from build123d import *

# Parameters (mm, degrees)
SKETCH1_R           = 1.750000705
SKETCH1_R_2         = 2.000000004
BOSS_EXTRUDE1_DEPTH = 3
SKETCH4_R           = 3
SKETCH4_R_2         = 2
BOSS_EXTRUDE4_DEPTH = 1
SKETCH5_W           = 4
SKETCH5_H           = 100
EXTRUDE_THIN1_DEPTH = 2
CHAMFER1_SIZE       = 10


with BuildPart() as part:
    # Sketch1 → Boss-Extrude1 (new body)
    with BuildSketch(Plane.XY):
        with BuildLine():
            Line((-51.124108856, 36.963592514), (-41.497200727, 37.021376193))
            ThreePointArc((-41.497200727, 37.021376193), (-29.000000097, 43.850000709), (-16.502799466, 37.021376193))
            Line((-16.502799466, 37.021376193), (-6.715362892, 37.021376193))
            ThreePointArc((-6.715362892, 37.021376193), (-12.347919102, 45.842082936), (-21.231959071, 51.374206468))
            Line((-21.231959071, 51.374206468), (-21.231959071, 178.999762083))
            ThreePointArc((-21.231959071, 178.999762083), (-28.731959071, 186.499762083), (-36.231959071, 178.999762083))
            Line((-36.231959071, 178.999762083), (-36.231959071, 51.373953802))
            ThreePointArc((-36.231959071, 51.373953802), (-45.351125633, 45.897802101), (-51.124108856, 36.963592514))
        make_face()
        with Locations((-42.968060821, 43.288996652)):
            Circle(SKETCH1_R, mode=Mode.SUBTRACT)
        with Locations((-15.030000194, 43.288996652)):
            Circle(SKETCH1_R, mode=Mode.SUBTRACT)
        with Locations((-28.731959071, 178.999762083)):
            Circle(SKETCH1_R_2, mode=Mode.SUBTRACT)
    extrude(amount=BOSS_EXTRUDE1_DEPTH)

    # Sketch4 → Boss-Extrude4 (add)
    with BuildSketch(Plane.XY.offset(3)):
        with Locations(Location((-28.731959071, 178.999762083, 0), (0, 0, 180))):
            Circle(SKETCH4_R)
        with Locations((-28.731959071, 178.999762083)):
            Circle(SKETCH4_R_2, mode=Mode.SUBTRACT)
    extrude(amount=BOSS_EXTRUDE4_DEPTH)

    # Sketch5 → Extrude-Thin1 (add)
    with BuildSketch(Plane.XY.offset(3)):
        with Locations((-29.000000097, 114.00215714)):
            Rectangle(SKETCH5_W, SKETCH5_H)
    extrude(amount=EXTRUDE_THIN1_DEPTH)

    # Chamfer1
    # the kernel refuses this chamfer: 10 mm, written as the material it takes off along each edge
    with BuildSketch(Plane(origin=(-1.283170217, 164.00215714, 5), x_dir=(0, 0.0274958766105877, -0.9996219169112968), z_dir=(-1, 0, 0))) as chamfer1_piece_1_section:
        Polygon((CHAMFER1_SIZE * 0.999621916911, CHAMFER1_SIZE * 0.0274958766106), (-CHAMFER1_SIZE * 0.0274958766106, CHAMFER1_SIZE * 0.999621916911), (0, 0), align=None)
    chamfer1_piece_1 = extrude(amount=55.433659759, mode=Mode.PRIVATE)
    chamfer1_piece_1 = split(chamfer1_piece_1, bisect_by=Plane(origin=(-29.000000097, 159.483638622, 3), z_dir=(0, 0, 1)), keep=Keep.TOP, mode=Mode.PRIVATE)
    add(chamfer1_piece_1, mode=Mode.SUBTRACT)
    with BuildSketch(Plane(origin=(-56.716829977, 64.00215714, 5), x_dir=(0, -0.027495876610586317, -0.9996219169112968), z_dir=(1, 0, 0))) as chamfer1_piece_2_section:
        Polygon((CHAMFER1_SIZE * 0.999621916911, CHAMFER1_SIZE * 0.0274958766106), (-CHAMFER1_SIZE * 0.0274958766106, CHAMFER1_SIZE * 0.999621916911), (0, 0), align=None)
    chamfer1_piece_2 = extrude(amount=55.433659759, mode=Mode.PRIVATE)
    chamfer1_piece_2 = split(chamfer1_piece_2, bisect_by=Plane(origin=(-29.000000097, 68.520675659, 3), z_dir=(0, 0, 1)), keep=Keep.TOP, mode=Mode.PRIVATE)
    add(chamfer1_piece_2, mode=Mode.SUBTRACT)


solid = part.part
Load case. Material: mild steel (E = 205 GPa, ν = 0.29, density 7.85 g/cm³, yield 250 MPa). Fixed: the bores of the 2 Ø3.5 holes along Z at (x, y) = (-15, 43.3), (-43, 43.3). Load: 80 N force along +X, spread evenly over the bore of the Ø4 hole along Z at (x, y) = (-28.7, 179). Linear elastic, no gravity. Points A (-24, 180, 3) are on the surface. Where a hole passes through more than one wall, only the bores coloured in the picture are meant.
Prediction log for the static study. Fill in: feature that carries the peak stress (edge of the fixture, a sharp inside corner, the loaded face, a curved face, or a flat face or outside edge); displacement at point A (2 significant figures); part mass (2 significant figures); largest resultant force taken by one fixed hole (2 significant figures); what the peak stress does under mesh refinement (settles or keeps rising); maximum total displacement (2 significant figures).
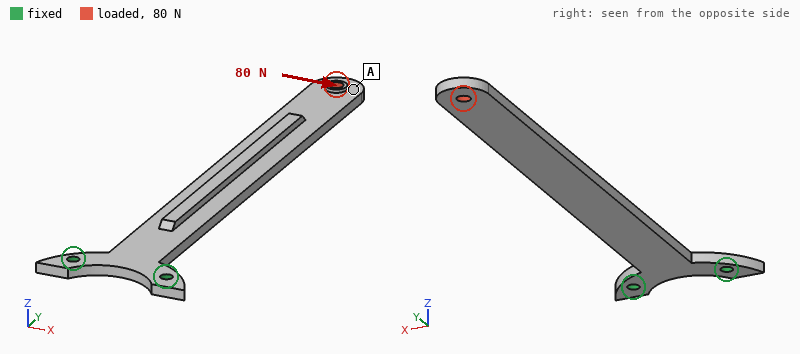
a sharp inside corner
0.38 mm
60 g
470 N
keeps rising
0.41 mm
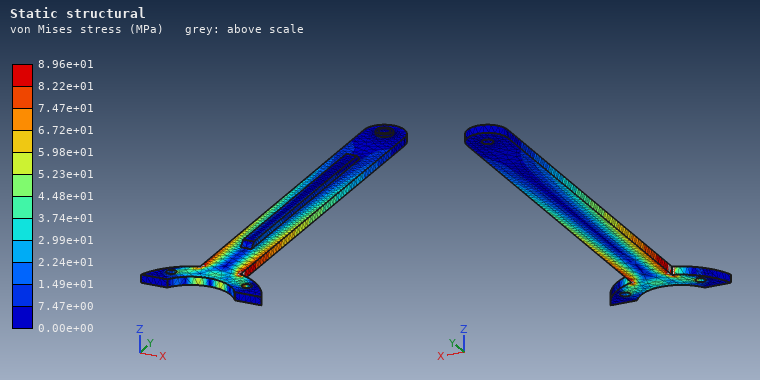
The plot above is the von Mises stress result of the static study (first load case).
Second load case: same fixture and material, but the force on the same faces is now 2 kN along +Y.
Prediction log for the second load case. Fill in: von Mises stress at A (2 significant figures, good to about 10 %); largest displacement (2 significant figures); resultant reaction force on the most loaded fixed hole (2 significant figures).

40 MPa
0.75 mm
1.3 kN
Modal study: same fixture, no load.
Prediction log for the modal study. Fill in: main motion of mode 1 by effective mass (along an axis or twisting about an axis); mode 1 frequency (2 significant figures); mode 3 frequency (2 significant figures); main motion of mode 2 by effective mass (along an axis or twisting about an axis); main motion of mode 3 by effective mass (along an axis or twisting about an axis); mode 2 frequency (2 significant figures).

along Z
130 Hz
980 Hz
along X
along Z
610 Hz
